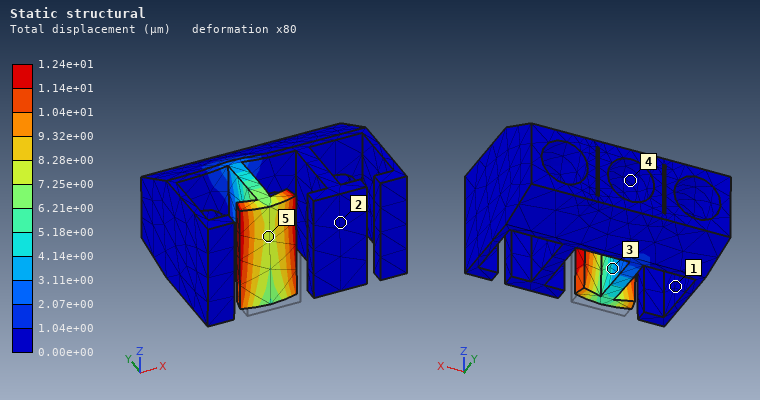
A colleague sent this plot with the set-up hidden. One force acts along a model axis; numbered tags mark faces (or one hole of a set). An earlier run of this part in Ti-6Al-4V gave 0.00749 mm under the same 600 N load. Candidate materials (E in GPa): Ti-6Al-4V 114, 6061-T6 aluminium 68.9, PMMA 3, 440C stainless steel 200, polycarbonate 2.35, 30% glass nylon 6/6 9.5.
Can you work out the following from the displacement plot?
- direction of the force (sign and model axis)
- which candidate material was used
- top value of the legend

+Y
6061-T6 aluminium
1.24e+01 µm
